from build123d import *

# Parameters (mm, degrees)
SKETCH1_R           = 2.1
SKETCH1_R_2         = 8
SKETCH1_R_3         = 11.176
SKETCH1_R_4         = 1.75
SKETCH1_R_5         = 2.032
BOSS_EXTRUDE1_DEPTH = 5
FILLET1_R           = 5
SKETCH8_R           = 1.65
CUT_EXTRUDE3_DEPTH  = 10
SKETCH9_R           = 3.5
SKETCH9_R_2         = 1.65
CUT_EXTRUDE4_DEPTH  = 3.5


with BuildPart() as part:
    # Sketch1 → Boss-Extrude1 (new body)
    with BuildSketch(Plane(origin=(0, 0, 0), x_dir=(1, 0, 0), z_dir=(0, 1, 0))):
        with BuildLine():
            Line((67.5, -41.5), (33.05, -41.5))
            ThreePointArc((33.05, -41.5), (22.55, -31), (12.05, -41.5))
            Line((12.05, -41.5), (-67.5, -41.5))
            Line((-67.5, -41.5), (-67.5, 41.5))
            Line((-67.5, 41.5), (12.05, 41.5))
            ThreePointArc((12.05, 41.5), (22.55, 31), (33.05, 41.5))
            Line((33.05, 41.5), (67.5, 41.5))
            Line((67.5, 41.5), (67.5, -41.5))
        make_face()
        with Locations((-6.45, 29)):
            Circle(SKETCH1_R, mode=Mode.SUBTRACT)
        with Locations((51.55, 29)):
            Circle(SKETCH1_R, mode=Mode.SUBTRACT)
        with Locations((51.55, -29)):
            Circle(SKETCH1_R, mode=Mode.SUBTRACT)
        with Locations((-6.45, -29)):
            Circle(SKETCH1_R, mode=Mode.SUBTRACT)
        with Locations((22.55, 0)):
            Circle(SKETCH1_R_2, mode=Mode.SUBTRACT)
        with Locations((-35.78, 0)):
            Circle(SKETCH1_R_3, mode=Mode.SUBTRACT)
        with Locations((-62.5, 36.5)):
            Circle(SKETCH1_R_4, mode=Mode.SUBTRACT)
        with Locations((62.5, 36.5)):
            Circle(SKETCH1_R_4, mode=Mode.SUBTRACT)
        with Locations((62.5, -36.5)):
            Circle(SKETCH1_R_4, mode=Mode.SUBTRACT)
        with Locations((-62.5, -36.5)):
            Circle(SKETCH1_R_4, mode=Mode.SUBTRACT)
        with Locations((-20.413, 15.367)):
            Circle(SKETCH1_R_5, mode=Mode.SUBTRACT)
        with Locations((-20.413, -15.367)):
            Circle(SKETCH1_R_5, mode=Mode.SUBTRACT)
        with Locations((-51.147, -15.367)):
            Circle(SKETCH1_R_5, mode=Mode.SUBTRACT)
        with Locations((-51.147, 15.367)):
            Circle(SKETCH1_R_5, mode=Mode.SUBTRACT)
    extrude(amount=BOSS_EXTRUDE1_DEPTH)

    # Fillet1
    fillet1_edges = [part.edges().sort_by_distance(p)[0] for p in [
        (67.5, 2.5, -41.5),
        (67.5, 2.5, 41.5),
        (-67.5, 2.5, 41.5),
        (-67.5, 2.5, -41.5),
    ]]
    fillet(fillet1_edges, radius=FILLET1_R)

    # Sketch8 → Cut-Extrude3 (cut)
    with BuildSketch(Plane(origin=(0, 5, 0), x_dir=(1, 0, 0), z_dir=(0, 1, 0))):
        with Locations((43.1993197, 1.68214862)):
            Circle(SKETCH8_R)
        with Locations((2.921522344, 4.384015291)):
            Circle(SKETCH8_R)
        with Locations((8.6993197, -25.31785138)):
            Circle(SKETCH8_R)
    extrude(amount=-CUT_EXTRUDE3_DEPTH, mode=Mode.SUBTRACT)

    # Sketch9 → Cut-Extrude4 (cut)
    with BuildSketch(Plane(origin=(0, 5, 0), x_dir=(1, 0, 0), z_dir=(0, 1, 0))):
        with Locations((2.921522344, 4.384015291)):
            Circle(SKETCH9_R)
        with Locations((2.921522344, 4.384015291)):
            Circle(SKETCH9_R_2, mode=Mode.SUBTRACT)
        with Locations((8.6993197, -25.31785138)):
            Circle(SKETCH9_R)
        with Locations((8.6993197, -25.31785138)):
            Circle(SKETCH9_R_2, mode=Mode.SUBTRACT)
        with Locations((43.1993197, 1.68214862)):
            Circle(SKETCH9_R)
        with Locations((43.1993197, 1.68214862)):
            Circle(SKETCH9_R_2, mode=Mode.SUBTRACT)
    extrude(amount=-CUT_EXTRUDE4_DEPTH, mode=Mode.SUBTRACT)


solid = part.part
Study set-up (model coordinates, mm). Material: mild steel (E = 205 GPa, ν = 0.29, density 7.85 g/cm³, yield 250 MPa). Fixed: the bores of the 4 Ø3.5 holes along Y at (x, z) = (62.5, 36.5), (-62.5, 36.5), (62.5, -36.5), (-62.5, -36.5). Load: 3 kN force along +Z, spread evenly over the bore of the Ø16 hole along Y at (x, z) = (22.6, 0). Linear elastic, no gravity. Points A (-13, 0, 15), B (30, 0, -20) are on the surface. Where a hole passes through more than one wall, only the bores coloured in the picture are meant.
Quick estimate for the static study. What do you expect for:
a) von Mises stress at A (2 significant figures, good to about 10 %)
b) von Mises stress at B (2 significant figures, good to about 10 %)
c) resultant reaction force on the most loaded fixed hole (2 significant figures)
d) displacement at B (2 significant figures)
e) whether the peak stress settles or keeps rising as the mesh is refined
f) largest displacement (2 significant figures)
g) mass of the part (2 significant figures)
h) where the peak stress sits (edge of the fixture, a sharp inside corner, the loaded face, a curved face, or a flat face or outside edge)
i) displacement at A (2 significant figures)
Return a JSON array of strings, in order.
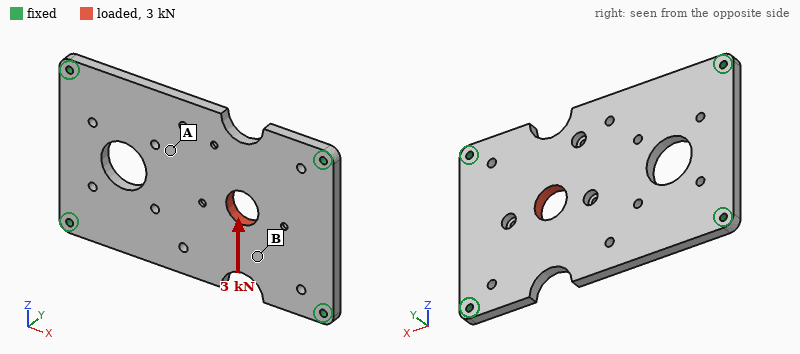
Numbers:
["4.6 MPa", "11 MPa", "1.3 kN", "4.0 µm", "keeps rising", "5.4 µm", "390 g", "edge of the fixture", "3.4 µm"]
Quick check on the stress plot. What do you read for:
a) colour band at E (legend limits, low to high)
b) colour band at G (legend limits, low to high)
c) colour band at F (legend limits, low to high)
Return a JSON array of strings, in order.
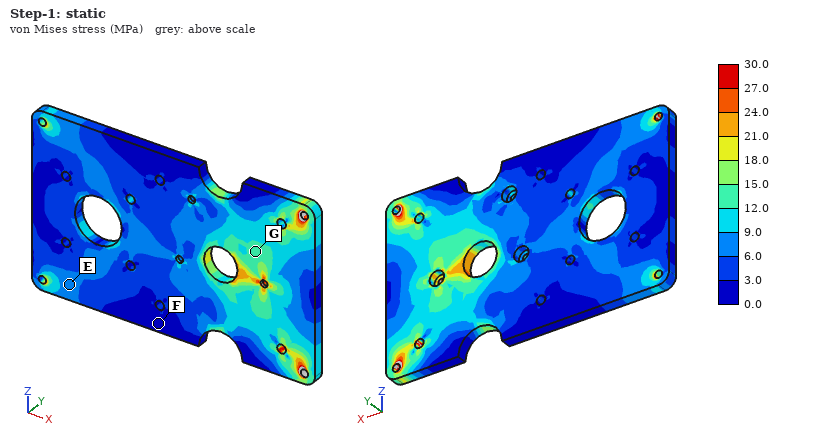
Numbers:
["6.0 to 9.0 MPa", "12.0 to 15.0 MPa", "0.0 to 3.0 MPa"]
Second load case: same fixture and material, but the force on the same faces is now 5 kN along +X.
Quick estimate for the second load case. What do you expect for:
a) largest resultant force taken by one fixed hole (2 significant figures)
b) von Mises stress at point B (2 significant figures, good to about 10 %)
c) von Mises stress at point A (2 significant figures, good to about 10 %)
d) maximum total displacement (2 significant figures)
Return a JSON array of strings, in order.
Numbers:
["1.6 kN", "8.8 MPa", "8.0 MPa", "5.5 µm"]
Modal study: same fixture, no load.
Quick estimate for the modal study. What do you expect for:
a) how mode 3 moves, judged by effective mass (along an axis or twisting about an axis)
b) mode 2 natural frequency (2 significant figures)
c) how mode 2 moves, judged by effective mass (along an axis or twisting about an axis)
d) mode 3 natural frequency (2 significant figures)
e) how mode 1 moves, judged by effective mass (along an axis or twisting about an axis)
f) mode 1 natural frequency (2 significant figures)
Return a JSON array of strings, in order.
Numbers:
["twisting about Z", "2200 Hz", "twisting about X", "3300 Hz", "along Y", "1300 Hz"]
